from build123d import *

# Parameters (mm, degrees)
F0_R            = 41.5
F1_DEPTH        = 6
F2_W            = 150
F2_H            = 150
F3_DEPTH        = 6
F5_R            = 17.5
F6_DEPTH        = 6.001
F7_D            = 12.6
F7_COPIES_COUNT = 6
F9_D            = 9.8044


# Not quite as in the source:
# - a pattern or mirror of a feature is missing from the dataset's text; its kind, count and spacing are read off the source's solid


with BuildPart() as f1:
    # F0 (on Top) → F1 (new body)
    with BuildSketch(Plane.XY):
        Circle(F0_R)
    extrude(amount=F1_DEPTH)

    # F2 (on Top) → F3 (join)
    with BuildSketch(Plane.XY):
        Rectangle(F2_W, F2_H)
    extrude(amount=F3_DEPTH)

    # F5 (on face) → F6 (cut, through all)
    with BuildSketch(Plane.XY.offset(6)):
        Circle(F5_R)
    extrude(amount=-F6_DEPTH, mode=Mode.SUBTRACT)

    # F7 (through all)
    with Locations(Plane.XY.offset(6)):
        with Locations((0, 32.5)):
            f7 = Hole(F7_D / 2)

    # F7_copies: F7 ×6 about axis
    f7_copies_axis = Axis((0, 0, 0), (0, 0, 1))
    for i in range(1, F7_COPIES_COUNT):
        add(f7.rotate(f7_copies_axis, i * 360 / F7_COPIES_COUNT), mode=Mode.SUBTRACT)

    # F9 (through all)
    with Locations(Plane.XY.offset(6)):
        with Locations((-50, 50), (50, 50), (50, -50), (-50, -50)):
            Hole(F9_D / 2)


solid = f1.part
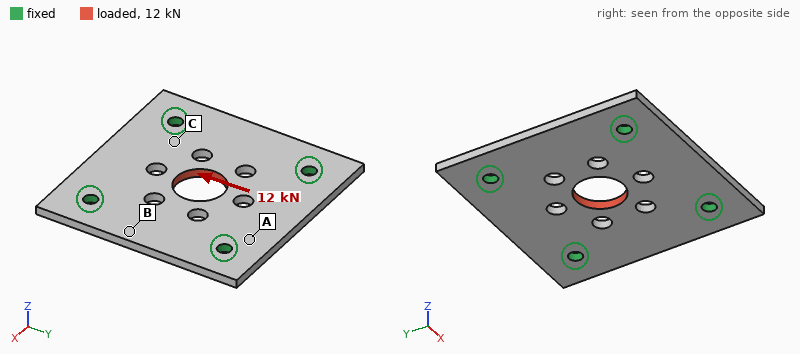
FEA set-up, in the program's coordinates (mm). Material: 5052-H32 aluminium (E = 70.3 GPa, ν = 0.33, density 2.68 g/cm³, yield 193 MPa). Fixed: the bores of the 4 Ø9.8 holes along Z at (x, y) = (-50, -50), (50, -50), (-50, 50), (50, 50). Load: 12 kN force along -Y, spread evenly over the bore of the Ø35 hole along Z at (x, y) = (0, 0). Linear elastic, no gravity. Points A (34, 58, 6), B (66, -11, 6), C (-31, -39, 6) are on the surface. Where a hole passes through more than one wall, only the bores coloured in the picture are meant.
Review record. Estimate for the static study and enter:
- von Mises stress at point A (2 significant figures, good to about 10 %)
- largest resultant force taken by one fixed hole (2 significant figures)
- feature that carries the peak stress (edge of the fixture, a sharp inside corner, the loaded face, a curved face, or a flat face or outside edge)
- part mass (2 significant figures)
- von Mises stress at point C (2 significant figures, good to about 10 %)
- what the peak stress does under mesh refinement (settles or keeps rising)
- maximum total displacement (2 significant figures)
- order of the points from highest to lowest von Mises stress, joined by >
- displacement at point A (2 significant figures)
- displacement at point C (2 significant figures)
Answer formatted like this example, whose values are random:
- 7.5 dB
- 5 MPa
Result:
- 11 MPa
- 3.2 kN
- edge of the fixture
- 330 g
- 18 MPa
- keeps rising
- 21 µm
- C > A > B
- 6.1 µm
- 7.2 µm
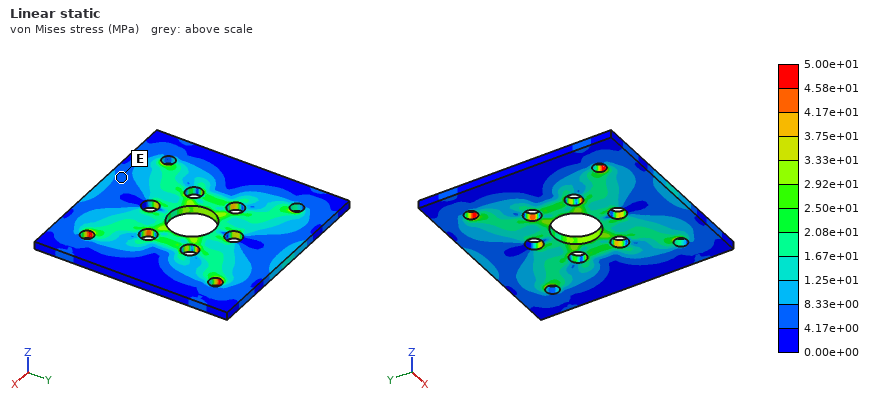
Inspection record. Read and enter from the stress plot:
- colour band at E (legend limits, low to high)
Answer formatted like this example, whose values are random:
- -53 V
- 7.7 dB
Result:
- 4.17e+00 to 8.33e+00 MPa
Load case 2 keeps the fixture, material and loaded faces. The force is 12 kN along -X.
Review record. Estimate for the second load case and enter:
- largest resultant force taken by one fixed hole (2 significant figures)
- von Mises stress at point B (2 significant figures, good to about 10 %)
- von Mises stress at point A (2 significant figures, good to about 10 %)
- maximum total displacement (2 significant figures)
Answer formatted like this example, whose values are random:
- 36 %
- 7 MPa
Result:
- 3.2 kN
- 8.4 MPa
- 5.5 MPa
- 21 µm
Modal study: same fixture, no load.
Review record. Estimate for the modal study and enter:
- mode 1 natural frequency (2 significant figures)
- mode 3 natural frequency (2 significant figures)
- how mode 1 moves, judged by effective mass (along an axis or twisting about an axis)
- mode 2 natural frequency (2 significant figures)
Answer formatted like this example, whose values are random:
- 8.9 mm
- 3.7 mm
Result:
- 2500 Hz
- 3300 Hz
- along Z
- 3200 Hz
